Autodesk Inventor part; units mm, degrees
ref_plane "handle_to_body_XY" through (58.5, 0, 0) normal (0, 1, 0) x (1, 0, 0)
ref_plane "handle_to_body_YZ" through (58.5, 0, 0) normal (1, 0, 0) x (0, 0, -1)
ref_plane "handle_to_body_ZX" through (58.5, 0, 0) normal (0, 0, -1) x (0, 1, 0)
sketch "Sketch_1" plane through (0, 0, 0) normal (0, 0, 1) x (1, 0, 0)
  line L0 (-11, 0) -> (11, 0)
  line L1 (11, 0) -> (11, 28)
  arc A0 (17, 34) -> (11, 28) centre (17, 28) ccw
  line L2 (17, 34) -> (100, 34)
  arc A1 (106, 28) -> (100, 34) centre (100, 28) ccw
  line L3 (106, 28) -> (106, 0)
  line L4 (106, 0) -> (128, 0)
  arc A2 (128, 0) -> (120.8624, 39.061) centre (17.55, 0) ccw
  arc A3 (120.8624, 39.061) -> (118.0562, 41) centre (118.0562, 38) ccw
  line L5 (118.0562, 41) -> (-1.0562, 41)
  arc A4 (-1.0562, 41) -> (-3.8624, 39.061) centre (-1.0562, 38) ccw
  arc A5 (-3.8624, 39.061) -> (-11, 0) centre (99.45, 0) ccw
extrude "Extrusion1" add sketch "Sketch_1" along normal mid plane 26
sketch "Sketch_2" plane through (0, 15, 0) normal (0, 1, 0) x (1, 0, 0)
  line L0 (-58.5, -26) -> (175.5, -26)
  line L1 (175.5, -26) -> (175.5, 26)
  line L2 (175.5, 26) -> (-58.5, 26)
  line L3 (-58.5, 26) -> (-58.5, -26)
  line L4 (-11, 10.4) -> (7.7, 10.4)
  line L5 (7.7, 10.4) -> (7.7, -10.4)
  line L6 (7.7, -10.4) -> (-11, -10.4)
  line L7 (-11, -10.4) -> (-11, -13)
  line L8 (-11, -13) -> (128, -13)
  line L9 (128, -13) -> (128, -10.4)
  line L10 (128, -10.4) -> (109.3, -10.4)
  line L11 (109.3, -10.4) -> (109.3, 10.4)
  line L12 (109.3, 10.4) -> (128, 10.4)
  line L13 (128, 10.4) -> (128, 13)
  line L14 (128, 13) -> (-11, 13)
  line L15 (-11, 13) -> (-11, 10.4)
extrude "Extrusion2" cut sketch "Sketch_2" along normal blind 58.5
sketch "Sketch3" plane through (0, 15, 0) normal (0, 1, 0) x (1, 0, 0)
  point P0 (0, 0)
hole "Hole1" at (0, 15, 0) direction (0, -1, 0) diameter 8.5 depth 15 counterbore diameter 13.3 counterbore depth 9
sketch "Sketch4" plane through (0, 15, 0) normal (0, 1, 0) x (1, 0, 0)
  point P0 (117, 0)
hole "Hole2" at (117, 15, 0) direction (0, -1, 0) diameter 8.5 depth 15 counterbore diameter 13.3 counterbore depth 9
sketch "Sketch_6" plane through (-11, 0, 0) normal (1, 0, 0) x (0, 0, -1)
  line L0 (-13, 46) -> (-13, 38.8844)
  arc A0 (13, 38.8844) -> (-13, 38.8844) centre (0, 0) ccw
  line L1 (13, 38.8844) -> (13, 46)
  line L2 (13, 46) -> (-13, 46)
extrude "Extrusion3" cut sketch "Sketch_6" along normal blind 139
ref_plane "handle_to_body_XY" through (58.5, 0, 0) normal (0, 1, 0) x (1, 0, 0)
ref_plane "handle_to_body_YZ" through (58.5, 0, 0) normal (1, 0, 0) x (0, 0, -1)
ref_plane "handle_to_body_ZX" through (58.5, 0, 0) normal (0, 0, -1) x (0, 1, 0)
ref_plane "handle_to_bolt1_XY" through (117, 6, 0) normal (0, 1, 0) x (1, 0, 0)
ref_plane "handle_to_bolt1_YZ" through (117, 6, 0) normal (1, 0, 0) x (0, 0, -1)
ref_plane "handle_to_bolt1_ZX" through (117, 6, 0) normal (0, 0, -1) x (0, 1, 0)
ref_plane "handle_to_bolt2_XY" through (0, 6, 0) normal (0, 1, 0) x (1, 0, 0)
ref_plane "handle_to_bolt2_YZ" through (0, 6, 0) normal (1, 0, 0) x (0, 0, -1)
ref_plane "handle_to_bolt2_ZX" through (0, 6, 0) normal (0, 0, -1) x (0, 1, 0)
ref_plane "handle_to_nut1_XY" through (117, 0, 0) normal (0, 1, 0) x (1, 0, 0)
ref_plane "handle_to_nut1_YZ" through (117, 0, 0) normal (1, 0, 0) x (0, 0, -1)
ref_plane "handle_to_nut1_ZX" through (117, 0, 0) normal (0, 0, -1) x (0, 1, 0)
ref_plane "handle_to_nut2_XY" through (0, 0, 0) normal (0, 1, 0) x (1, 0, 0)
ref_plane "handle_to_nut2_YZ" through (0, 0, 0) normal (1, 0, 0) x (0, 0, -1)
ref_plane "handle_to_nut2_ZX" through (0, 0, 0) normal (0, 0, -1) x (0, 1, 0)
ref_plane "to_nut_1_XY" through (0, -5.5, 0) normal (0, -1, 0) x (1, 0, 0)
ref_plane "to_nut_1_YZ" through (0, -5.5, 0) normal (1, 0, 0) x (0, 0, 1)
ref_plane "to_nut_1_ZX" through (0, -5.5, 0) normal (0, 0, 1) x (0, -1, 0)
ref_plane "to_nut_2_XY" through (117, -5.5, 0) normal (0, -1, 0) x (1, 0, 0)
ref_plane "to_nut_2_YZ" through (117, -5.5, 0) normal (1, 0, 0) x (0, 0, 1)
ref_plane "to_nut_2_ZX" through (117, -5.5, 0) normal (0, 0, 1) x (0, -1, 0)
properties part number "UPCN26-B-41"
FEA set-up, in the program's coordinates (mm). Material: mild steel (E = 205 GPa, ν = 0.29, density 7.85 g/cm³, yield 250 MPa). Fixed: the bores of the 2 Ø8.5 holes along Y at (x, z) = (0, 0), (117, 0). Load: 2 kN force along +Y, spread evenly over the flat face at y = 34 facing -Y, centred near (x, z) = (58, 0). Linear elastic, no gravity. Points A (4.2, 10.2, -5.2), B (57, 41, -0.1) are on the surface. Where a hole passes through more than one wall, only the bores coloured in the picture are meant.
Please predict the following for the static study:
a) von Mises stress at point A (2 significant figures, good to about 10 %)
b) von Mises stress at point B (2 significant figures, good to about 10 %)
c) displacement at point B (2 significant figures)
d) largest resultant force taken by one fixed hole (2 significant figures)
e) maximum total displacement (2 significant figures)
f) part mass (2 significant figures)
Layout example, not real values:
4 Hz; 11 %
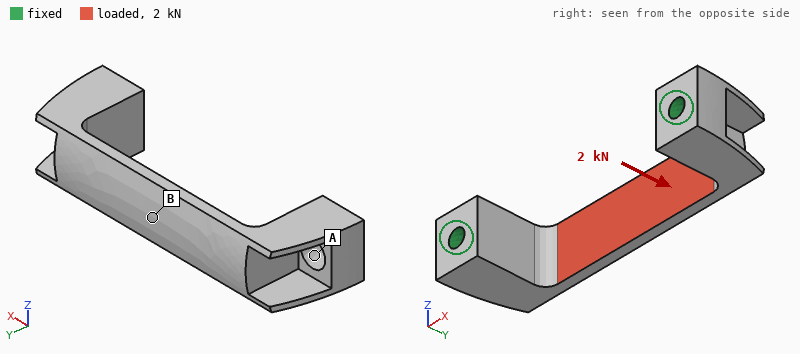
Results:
15 MPa; 76 MPa; 66 µm; 1.3 kN; 68 µm; 300 g
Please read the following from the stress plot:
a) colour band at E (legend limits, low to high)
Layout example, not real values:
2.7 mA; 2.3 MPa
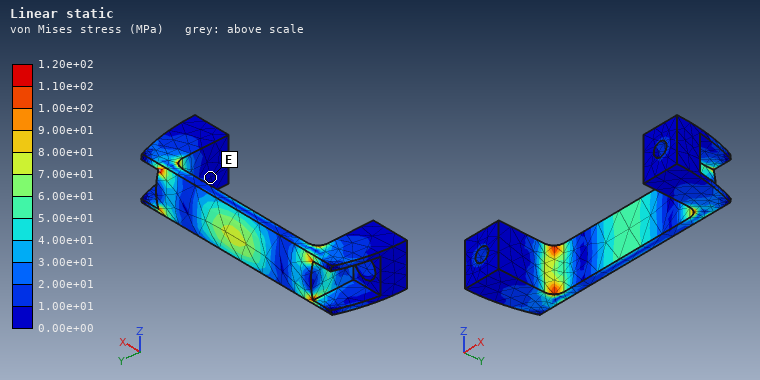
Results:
0.00e+00 to 1.00e+01 MPa
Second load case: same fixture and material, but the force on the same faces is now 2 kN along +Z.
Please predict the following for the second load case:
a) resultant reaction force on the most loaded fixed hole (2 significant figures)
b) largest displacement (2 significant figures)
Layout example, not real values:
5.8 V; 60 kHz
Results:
1.0 kN; 36 µm
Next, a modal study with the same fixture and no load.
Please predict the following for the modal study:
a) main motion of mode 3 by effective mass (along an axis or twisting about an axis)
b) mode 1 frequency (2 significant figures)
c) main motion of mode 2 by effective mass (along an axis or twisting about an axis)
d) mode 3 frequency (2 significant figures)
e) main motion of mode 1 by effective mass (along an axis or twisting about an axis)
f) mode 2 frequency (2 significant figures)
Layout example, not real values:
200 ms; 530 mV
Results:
along X; 3000 Hz; along Z; 3700 Hz; along Y; 3200 Hz
